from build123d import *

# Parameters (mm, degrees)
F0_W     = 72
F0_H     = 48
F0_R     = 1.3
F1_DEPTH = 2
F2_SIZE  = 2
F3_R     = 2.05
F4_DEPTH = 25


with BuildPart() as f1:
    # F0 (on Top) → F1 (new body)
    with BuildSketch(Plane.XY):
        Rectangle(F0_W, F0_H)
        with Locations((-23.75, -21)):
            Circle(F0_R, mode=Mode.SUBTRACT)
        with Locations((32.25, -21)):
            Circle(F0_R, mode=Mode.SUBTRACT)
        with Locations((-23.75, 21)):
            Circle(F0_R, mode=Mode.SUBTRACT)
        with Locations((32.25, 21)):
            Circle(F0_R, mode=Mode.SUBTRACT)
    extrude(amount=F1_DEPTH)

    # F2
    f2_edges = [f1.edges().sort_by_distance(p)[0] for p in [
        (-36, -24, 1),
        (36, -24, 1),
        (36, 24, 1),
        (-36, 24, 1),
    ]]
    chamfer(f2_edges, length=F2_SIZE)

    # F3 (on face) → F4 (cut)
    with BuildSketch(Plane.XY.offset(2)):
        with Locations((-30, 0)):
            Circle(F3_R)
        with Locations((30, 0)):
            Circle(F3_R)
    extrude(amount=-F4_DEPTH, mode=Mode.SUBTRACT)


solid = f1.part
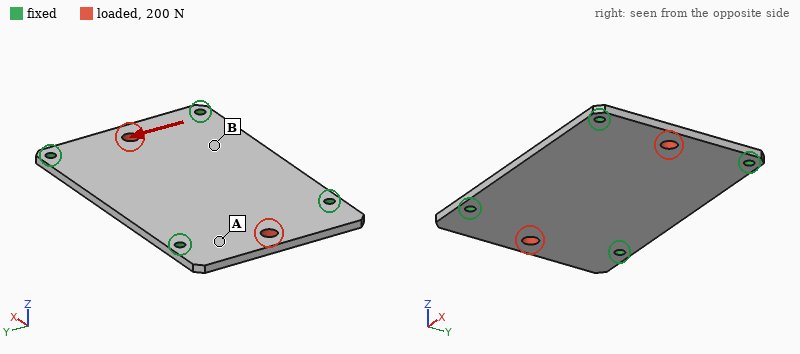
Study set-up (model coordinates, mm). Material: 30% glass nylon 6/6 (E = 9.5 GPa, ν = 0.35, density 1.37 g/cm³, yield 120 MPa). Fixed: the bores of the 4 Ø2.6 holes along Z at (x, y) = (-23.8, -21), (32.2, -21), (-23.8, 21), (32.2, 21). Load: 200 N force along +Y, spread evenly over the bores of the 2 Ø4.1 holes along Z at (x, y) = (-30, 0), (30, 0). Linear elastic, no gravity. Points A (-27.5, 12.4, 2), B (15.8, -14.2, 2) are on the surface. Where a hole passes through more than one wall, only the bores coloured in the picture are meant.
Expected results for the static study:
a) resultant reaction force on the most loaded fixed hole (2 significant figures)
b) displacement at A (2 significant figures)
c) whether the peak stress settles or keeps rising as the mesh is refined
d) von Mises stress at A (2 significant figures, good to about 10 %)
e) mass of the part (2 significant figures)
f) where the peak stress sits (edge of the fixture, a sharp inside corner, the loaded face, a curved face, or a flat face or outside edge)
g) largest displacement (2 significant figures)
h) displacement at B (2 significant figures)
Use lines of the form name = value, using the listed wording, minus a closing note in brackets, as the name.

resultant reaction force on the most loaded fixed hole = 53 N
displacement at A = 2.9 µm
whether the peak stress settles or keeps rising as the mesh is refined = keeps rising
von Mises stress at A = 2.2 MPa
mass of the part = 9.3 g
where the peak stress sits = edge of the fixture
largest displacement = 6.7 µm
displacement at B = 3.1 µm
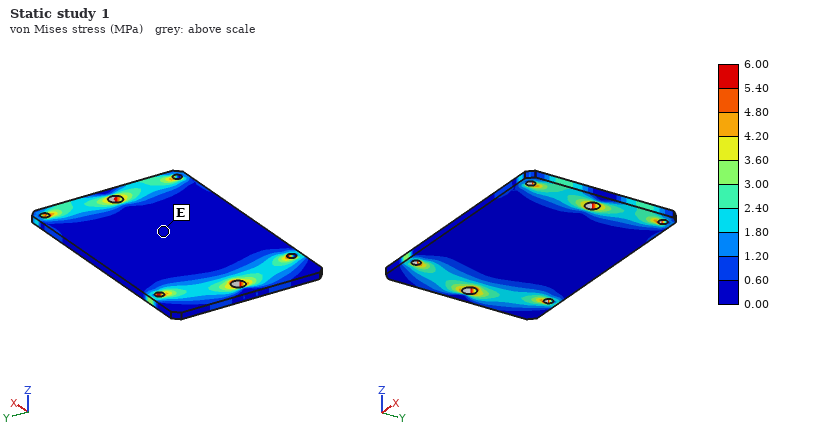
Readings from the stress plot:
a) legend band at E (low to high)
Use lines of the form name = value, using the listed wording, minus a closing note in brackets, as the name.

legend band at E = 0.00 to 0.60 MPa
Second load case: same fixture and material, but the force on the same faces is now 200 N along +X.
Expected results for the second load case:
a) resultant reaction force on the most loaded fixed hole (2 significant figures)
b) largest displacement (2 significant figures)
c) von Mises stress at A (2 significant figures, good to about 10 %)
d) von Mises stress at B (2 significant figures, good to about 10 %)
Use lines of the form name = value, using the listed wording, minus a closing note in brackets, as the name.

resultant reaction force on the most loaded fixed hole = 56 N
largest displacement = 12 µm
von Mises stress at A = 1.5 MPa
von Mises stress at B = 1.3 MPa
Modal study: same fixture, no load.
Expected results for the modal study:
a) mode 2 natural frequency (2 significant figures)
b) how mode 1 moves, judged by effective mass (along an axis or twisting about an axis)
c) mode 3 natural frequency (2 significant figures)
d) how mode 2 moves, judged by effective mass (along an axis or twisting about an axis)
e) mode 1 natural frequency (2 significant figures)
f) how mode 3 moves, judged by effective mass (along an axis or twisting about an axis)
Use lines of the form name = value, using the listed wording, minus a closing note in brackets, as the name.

mode 2 natural frequency = 2200 Hz
how mode 1 moves, judged by effective mass = along Z
mode 3 natural frequency = 2600 Hz
how mode 2 moves, judged by effective mass = twisting about X
mode 1 natural frequency = 1400 Hz
how mode 3 moves, judged by effective mass = along Z
